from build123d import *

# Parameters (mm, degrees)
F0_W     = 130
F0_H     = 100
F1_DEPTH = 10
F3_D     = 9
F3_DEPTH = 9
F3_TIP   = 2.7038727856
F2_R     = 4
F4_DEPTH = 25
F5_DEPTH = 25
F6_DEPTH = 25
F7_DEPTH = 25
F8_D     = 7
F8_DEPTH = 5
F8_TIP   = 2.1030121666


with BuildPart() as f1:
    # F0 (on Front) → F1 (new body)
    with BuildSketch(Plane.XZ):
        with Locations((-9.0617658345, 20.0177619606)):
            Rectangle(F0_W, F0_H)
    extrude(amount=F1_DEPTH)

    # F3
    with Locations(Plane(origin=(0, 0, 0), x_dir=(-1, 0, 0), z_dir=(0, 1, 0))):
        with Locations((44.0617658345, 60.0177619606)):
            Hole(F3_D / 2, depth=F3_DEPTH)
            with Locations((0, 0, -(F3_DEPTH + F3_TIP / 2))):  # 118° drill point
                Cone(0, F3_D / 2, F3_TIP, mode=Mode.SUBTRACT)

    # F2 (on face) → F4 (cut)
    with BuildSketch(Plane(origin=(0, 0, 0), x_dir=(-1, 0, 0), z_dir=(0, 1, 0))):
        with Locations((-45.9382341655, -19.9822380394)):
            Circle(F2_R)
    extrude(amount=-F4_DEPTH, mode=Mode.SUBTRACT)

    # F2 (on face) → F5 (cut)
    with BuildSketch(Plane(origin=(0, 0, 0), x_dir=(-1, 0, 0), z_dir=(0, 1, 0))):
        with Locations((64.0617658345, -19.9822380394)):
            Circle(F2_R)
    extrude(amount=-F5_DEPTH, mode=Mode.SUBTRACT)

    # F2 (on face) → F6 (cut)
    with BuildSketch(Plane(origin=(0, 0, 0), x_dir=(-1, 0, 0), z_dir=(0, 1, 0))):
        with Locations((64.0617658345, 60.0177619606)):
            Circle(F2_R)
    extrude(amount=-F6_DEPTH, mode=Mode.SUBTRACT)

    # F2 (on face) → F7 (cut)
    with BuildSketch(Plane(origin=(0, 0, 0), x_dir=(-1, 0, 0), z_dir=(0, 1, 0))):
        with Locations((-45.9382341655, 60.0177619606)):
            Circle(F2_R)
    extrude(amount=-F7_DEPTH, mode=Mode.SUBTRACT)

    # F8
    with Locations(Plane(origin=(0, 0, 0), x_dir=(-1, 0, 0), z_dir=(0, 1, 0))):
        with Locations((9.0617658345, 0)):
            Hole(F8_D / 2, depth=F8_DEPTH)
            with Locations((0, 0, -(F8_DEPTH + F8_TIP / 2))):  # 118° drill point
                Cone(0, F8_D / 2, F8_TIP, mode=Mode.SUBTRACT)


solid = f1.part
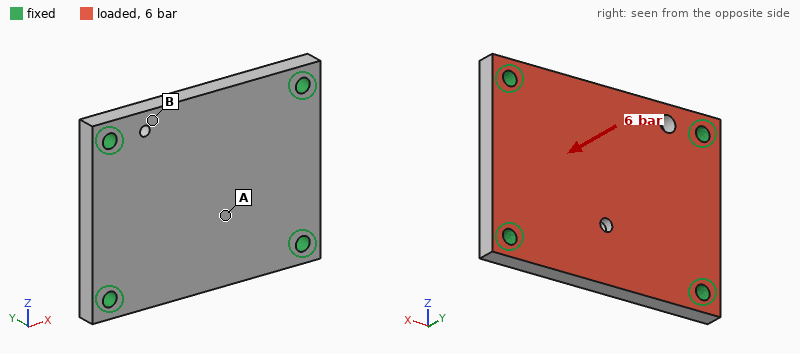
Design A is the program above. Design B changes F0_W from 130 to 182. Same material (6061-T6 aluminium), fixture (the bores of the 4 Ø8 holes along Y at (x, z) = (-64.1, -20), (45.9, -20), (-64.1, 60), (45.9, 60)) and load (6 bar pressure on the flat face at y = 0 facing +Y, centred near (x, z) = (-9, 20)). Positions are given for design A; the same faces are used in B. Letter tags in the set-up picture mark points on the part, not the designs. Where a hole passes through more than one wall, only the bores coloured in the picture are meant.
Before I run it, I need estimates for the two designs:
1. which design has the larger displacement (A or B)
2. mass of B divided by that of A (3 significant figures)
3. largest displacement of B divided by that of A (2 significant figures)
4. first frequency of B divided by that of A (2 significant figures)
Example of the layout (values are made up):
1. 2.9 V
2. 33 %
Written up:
1. A
2. 1.41
3. 0.87
4. 1.00
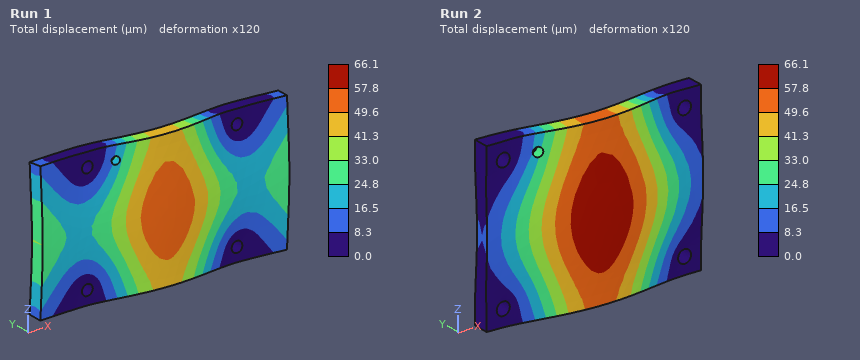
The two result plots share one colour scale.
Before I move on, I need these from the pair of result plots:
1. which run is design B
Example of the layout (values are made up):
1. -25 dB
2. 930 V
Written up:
1. Run 1
